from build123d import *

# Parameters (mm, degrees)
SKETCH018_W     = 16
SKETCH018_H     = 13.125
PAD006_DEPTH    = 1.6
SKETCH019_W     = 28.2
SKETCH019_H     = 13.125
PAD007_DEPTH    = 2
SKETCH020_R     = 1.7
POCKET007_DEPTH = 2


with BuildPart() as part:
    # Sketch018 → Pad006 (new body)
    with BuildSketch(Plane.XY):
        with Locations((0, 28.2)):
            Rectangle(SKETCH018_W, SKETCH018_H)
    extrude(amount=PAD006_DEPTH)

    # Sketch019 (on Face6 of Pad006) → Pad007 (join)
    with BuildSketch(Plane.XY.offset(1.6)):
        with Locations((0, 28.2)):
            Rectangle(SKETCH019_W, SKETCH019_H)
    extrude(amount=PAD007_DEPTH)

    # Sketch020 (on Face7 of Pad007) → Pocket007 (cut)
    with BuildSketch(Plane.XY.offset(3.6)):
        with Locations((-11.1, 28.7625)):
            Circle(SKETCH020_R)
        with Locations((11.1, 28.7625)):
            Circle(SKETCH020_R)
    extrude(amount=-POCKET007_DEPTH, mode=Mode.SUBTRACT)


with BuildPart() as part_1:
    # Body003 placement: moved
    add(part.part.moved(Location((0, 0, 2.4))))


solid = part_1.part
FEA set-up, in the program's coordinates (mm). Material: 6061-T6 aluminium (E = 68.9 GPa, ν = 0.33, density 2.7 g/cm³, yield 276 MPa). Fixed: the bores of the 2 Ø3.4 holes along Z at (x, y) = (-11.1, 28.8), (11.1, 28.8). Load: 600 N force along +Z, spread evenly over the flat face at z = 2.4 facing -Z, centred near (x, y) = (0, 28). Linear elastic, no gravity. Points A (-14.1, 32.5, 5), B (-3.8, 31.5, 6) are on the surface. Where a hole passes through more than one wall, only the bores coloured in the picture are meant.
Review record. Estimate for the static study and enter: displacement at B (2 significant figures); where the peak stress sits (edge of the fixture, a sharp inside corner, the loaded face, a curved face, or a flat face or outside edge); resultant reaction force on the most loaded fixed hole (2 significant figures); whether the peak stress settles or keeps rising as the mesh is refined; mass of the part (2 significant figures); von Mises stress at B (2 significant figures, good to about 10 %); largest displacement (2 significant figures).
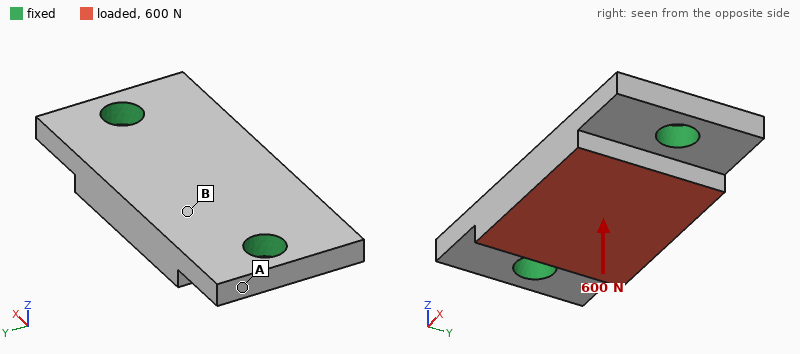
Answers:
10 µm
edge of the fixture
390 N
keeps rising
2.8 g
21 MPa
19 µm
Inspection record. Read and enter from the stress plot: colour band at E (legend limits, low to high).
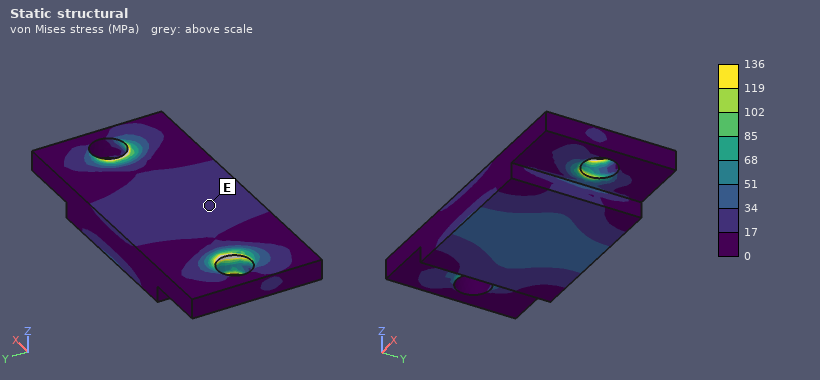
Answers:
17 to 34 MPa
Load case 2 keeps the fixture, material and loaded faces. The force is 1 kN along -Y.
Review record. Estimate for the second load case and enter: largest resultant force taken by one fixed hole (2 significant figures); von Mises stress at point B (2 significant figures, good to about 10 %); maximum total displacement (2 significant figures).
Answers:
500 N
25 MPa
36 µm
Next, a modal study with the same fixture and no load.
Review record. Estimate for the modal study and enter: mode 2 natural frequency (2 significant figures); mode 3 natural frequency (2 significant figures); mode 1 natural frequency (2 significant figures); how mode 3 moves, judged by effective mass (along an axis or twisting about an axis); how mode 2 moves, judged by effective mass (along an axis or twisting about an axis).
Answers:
26 kHz
46 kHz
21 kHz
along Y
along Z
